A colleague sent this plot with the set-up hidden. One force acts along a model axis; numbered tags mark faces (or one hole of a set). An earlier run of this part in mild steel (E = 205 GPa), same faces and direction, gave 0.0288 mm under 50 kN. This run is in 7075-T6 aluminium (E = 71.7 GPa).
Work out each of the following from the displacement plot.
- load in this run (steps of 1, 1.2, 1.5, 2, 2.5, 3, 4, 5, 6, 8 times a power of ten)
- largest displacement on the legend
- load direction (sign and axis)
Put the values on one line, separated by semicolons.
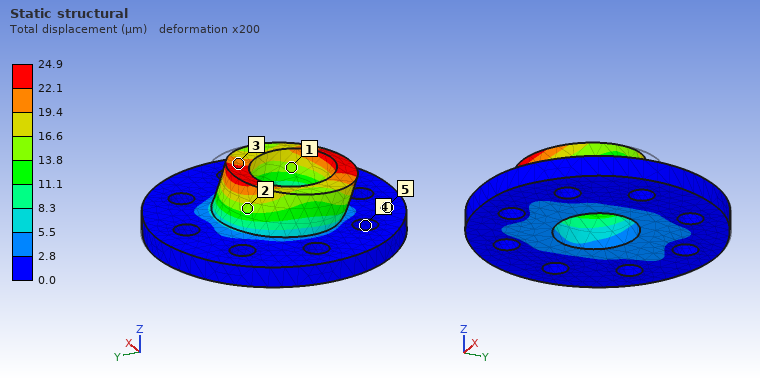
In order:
15 kN; 24.9 µm; -Y
